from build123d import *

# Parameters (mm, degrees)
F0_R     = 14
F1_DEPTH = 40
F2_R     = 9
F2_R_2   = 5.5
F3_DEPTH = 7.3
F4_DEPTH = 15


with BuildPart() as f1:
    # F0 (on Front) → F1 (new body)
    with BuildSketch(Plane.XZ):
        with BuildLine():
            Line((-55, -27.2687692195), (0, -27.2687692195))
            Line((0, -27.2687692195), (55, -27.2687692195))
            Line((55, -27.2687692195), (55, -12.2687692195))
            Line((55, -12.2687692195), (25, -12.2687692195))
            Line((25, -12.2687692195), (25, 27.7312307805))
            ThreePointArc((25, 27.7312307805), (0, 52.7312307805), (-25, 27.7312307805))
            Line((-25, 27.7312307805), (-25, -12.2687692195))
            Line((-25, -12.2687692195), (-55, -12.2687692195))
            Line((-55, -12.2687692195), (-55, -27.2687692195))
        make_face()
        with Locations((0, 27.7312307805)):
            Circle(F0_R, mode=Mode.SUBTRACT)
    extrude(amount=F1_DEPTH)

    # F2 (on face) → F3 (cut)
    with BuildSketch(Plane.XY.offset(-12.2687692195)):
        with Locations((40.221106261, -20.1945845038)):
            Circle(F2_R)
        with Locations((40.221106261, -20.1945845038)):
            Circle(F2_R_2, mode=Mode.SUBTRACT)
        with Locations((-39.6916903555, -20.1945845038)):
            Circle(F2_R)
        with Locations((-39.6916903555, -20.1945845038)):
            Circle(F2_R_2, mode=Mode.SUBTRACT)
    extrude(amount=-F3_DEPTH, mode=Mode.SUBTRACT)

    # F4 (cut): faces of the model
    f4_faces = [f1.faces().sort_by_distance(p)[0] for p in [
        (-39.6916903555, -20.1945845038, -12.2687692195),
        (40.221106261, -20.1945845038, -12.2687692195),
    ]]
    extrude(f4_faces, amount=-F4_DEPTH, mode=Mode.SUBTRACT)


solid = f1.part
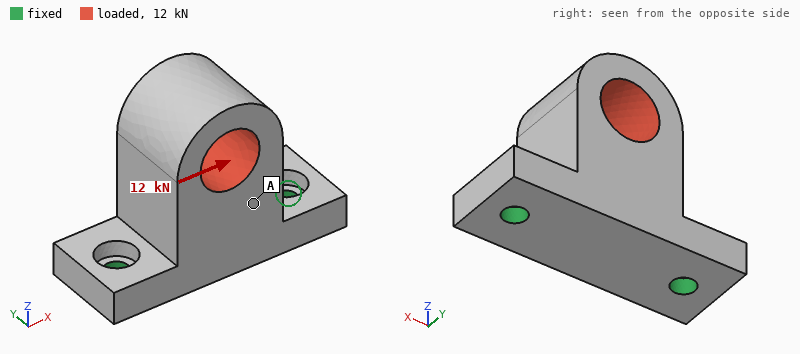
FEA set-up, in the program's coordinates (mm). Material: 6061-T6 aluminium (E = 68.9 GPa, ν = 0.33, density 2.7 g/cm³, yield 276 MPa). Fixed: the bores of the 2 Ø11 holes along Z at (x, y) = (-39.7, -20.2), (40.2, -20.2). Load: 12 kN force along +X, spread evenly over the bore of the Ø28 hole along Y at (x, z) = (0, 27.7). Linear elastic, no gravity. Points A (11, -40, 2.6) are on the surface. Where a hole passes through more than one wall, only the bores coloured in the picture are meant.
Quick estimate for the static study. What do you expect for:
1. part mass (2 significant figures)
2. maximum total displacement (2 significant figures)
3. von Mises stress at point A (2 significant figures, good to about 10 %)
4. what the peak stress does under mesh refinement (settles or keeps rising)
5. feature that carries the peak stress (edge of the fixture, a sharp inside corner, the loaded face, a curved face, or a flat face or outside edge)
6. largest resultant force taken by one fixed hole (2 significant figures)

420 g
0.12 mm
15 MPa
keeps rising
edge of the fixture
11 kN
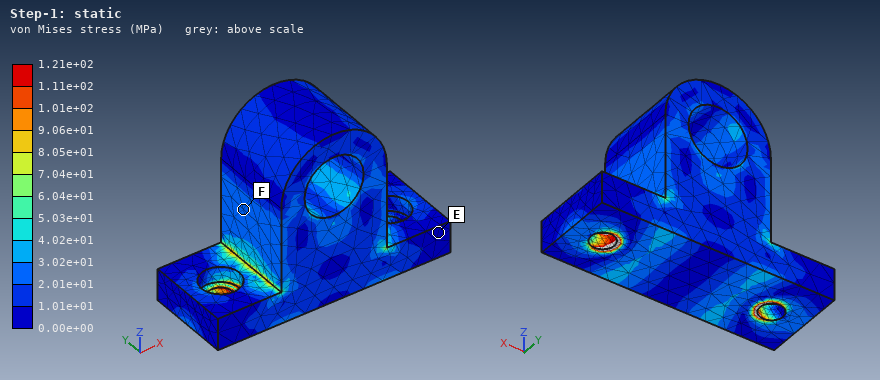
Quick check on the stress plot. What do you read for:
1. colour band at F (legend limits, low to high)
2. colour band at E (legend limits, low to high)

2.01e+01 to 3.02e+01 MPa
0.00e+00 to 1.01e+01 MPa
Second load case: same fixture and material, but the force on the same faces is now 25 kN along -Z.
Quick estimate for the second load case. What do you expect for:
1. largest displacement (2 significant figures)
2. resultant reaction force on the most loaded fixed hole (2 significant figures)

68 µm
15 kN
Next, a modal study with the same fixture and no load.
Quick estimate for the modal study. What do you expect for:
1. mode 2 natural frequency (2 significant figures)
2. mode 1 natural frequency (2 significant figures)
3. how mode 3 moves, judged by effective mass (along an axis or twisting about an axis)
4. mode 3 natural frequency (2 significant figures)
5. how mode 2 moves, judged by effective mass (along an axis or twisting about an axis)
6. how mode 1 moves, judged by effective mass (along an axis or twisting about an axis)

4500 Hz
1600 Hz
along Z
6000 Hz
along X
along Y
